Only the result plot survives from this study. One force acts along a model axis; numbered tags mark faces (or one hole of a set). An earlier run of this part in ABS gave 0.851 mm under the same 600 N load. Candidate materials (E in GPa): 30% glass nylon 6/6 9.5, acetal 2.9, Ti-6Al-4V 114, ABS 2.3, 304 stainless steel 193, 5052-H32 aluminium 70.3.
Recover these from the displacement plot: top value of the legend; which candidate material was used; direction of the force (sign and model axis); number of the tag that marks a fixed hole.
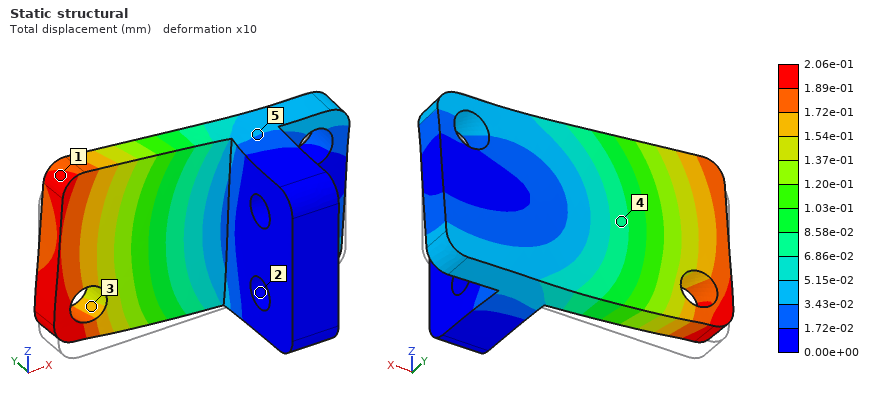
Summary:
2.06e-01 mm
30% glass nylon 6/6
+Z
2
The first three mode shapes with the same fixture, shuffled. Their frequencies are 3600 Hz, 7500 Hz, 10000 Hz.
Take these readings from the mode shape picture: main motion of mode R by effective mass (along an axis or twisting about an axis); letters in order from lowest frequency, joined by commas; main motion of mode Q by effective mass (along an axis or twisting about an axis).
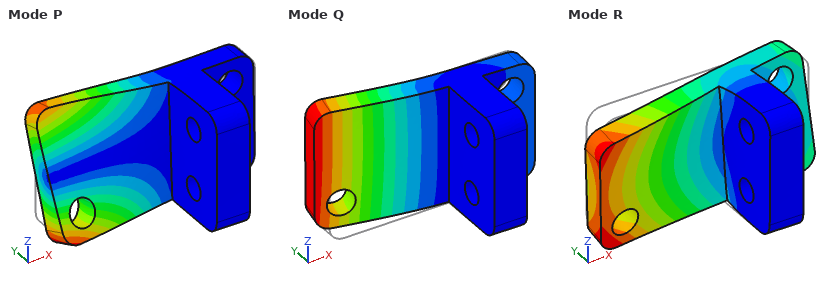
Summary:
along Z
Q, R, P
along Y
